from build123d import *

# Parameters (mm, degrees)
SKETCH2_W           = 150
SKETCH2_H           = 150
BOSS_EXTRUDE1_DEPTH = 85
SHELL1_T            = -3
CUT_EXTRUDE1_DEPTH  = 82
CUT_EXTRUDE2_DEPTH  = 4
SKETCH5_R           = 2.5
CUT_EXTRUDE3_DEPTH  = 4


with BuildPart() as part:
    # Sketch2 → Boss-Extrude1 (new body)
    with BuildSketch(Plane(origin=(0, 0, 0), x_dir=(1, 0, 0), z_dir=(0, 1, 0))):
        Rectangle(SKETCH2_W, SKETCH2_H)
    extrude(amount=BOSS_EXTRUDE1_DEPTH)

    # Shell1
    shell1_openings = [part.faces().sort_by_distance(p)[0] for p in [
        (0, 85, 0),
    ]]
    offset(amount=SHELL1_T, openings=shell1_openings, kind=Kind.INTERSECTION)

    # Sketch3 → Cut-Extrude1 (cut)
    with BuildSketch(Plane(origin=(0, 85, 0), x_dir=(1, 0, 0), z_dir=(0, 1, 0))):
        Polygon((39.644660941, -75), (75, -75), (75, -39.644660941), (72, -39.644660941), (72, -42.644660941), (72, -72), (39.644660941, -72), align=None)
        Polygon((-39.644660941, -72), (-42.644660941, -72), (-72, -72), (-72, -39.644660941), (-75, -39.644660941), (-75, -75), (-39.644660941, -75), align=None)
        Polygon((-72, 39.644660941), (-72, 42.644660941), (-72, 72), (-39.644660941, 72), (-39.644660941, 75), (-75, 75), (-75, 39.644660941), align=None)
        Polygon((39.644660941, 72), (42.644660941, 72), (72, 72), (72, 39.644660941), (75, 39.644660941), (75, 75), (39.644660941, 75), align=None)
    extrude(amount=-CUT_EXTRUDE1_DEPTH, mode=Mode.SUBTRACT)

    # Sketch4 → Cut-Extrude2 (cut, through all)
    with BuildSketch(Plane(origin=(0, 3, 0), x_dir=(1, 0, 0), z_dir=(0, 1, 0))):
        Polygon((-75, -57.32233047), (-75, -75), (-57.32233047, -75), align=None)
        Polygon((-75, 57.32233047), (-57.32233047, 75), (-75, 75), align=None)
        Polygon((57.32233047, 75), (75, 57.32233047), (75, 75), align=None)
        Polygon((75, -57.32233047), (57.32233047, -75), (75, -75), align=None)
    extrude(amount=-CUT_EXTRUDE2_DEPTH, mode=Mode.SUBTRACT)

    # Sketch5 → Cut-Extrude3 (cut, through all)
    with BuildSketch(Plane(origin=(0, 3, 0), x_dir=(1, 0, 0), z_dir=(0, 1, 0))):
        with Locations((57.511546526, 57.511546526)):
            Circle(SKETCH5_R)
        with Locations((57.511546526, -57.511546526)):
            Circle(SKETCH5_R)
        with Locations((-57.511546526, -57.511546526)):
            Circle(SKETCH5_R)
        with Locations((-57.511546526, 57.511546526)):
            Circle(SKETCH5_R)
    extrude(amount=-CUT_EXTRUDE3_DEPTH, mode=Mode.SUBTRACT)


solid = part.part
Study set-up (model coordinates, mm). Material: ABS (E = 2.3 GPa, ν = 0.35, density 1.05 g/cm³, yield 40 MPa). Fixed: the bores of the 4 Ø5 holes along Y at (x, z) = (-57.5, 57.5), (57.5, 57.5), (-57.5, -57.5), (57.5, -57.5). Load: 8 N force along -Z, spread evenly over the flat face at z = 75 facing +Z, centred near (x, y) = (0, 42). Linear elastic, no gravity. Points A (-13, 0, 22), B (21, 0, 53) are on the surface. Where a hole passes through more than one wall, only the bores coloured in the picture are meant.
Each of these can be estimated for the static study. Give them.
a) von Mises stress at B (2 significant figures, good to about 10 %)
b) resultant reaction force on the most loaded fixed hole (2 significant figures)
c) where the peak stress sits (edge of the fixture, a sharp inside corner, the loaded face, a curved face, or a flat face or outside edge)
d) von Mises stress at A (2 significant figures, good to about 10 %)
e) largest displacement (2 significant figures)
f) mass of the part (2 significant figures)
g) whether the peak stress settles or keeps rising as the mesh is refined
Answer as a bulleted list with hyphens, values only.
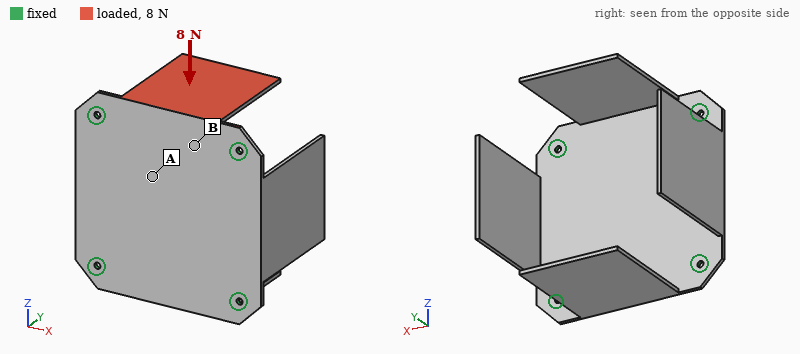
- 1.1 MPa
- 2.7 N
- edge of the fixture
- 0.41 MPa
- 2.4 mm
- 150 g
- keeps rising
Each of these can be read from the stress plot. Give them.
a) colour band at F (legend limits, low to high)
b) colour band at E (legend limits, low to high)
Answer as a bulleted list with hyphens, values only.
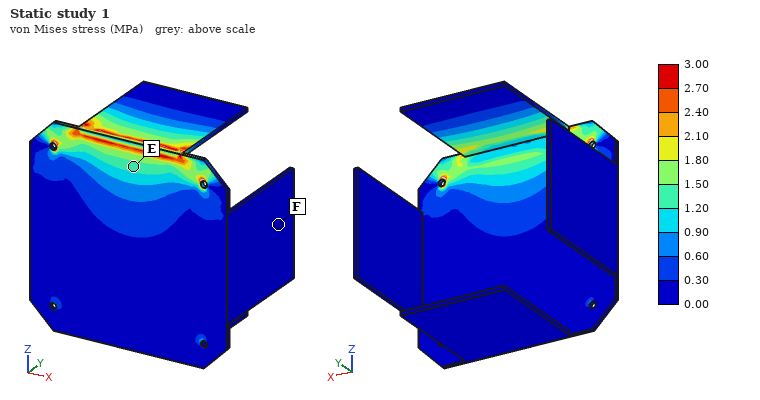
- 0.00 to 0.30 MPa
- 1.20 to 1.50 MPa
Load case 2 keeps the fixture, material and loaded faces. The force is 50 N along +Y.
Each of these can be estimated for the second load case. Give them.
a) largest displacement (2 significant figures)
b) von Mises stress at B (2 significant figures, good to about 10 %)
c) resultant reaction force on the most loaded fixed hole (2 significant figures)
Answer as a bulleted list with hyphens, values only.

- 2.3 mm
- 1.6 MPa
- 29 N
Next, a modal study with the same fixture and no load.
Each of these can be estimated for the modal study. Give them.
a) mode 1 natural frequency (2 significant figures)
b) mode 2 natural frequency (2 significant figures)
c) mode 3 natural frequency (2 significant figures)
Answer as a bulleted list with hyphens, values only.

- 72 Hz
- 79 Hz
- 79 Hz
